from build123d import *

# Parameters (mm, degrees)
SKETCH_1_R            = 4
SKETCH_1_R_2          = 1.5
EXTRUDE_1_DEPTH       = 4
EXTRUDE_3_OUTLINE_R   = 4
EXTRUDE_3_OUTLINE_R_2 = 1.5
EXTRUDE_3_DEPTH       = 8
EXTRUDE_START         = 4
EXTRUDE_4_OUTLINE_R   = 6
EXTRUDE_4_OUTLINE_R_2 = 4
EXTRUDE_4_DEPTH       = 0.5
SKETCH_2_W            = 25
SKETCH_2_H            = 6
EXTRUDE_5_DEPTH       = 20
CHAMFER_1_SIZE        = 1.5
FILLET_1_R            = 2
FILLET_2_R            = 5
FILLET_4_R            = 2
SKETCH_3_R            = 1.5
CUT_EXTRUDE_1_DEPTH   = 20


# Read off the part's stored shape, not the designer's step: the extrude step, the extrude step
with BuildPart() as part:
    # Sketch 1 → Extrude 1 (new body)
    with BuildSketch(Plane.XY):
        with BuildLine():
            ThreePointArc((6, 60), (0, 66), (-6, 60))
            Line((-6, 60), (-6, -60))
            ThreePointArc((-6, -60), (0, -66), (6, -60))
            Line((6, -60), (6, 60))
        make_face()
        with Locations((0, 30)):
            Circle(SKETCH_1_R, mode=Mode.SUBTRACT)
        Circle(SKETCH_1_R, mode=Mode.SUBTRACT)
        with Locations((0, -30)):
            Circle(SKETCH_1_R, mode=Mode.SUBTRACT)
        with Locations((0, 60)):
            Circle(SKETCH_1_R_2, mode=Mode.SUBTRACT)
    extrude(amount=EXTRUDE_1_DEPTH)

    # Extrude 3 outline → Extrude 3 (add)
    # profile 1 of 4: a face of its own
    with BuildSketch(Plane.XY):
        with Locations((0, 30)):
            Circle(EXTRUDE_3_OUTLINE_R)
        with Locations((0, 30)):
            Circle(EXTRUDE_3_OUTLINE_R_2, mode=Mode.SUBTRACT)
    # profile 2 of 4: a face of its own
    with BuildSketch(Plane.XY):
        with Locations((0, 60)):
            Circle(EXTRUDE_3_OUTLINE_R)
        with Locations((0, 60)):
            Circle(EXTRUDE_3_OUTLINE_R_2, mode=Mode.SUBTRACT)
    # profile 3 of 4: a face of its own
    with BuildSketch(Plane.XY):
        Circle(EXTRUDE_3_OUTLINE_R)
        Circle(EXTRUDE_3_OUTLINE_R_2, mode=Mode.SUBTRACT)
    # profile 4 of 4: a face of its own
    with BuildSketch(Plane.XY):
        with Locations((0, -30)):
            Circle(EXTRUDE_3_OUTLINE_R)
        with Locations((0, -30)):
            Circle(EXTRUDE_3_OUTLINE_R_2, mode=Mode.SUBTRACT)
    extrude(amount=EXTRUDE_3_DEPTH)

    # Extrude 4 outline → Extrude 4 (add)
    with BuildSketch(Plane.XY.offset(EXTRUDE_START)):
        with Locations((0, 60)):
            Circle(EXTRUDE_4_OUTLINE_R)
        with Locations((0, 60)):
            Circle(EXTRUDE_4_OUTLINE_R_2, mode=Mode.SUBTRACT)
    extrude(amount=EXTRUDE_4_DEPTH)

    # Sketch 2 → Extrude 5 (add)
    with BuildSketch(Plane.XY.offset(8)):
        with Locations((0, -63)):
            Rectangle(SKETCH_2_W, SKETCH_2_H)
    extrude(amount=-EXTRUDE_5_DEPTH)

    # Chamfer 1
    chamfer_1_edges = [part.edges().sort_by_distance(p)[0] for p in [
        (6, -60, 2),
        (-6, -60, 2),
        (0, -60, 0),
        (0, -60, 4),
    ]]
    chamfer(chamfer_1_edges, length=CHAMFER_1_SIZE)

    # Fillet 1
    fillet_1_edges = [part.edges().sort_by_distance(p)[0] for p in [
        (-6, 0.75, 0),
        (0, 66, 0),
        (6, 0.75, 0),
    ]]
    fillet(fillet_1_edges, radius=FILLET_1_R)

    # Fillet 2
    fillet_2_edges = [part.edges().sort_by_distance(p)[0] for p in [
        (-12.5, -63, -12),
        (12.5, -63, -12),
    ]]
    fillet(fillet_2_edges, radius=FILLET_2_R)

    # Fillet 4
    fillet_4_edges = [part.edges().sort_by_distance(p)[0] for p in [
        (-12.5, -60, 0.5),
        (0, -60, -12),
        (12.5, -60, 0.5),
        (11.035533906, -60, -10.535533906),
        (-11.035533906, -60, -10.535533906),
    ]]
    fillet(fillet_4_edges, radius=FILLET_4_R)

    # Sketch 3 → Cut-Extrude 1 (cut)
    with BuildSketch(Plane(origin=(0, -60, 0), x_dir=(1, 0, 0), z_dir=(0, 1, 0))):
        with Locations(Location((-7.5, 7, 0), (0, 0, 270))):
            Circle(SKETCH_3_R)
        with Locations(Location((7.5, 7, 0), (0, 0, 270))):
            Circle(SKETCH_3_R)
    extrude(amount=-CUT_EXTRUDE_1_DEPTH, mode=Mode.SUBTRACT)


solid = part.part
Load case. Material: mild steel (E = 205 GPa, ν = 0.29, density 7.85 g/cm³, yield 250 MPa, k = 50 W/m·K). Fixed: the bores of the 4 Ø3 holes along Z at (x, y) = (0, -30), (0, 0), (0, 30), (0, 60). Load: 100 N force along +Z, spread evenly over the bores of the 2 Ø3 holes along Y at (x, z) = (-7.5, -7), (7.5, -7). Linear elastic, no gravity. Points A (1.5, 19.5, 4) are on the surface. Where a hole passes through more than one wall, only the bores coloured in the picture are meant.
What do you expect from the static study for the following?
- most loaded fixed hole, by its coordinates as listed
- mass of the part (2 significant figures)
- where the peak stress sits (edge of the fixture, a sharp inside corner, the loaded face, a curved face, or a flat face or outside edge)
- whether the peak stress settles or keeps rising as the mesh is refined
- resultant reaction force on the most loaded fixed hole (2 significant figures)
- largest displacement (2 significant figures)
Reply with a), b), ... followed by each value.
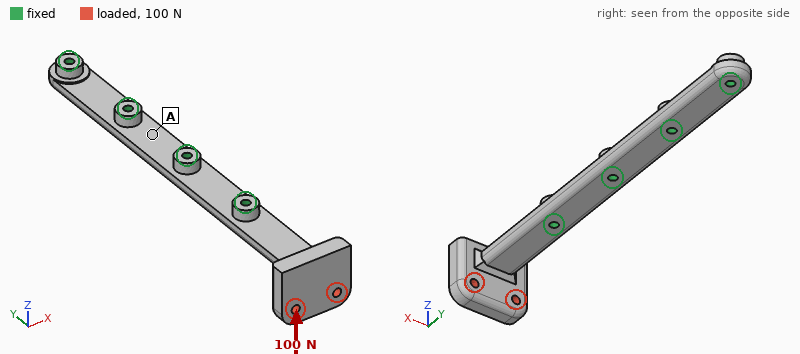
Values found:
a) (0, -30)
b) 72 g
c) edge of the fixture
d) keeps rising
e) 100 N
f) 0.11 mm
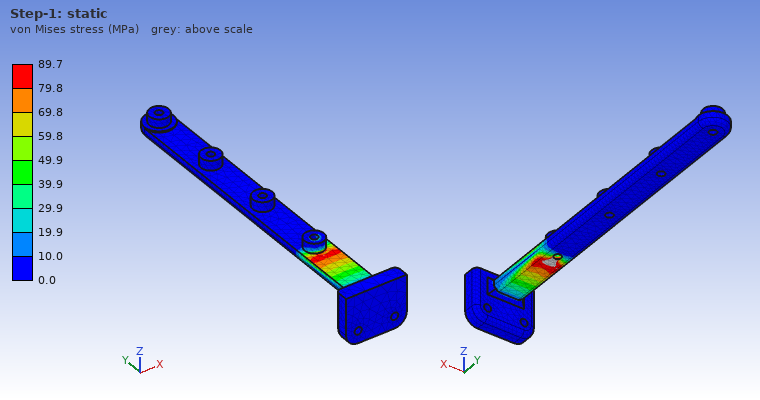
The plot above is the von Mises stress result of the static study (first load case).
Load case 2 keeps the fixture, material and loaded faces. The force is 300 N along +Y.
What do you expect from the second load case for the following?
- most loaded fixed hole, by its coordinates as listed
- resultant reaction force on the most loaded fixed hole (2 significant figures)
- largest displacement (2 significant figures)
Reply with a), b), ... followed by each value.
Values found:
a) (0, -30)
b) 280 N
c) 0.16 mm
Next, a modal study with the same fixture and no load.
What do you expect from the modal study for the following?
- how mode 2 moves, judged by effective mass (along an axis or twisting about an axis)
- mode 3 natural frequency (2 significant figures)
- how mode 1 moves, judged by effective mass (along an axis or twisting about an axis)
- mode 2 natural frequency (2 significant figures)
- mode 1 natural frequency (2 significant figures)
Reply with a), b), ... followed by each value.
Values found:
a) along X
b) 3100 Hz
c) along Z
d) 2200 Hz
e) 1100 Hz
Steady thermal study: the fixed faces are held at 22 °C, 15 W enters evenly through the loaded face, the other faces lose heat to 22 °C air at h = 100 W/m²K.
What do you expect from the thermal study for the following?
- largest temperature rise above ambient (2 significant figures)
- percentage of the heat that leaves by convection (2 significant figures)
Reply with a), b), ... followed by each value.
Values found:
a) 77 K
b) 75 %
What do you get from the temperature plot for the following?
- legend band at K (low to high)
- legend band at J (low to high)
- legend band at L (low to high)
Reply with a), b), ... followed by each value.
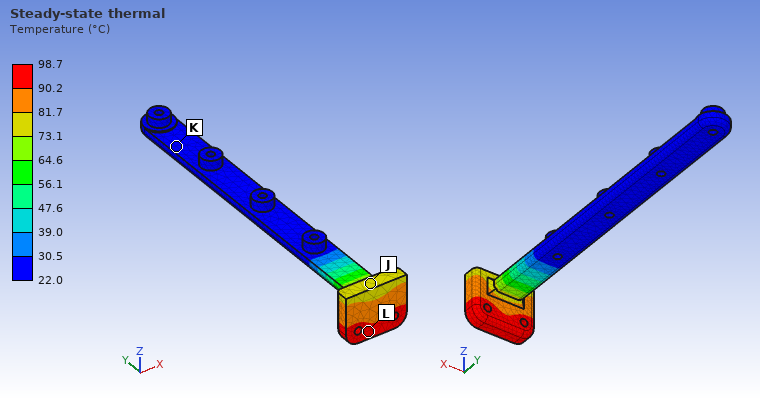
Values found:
a) 22.0 to 30.5 °C
b) 73.1 to 81.7 °C
c) 90.2 to 98.7 °C
